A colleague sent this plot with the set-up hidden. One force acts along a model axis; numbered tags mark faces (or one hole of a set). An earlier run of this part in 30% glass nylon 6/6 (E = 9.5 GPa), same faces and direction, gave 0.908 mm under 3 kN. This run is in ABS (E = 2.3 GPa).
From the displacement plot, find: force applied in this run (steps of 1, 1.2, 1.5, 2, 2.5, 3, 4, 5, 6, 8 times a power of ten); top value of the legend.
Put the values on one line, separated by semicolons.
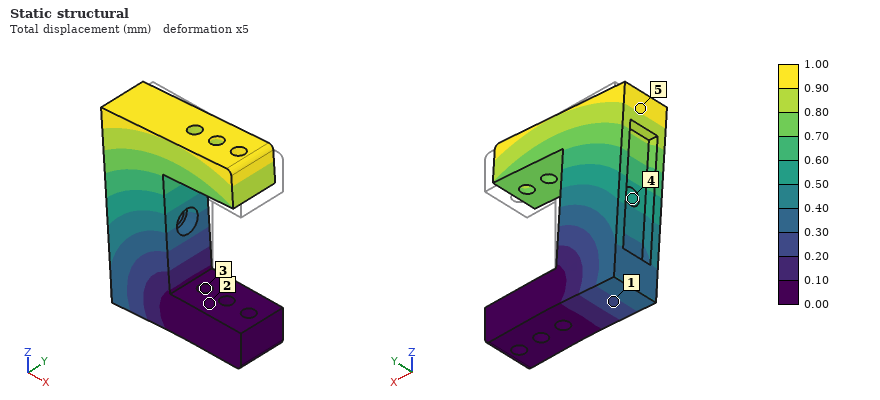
800 N; 1.00 mm
